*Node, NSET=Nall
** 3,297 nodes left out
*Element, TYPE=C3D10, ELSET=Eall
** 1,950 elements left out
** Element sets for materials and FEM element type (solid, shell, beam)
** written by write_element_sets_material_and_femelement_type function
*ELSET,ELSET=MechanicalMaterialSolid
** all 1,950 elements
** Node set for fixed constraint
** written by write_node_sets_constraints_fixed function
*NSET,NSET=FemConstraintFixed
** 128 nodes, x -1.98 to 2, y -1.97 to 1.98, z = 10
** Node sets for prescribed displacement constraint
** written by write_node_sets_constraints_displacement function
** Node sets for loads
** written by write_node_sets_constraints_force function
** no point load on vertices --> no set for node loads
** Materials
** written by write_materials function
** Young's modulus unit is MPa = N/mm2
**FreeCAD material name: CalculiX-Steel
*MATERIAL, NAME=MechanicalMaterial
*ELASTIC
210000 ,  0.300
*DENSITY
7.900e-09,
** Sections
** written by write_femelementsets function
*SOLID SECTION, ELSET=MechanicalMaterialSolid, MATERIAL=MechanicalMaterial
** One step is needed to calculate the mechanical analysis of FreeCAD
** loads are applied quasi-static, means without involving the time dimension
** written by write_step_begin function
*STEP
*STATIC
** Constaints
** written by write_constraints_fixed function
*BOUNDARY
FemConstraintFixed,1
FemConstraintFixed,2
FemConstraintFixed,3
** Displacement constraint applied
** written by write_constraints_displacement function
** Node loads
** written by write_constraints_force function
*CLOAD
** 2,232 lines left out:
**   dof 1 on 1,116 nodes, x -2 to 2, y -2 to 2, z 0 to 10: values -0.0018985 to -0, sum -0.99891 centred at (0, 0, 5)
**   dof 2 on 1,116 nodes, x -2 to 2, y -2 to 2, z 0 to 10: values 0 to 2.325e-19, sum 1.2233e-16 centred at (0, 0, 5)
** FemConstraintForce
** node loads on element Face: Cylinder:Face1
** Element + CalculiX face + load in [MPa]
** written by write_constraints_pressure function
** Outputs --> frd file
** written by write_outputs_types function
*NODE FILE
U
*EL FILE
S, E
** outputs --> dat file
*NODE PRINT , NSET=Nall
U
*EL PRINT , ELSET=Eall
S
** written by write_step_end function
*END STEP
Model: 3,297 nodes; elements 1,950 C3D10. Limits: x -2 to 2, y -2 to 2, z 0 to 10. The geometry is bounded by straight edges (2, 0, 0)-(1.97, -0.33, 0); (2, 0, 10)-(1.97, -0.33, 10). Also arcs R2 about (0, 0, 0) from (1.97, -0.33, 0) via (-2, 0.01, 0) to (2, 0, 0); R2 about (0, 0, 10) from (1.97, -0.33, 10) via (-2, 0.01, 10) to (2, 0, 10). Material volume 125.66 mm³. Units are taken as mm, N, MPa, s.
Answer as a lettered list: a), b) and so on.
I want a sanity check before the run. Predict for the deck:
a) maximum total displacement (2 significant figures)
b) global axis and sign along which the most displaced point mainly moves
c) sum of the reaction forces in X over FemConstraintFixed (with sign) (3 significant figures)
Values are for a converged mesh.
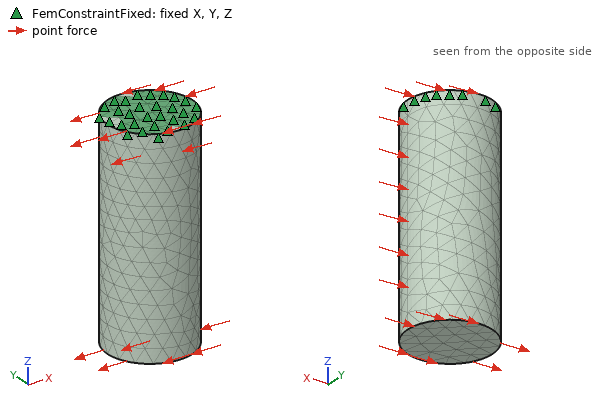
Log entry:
a) 5.4e-05 mm
b) -X
c) 0.999 N
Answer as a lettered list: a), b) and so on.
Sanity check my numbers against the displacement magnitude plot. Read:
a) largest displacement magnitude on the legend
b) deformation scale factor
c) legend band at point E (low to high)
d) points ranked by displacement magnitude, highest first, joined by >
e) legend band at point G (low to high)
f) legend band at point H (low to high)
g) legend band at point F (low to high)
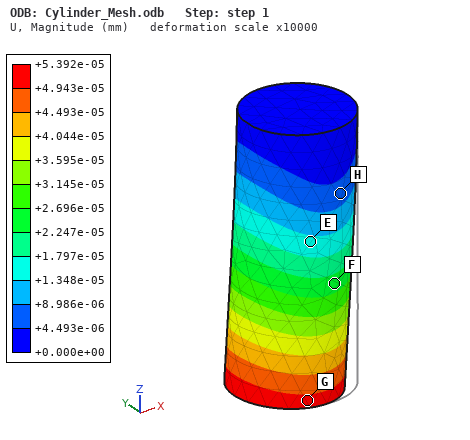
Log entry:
a) +5.392e-05 mm
b) 10000
c) +1.348e-05 to +1.797e-05 mm
d) G > F > E > H
e) +4.943e-05 to +5.392e-05 mm
f) +4.493e-06 to +8.986e-06 mm
g) +2.247e-05 to +2.696e-05 mm
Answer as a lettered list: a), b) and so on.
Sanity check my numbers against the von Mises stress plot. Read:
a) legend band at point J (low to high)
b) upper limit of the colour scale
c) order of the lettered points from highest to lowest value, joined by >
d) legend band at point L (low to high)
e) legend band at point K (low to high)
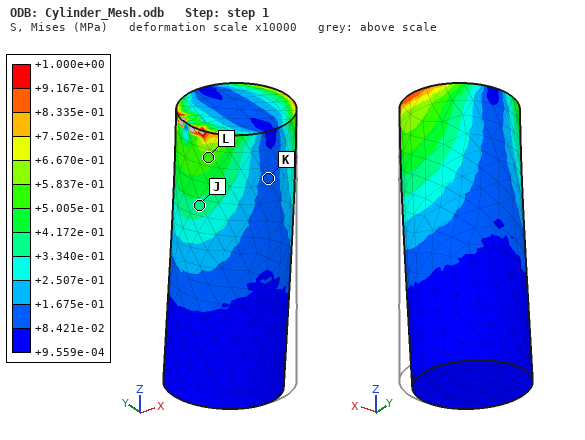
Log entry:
a) +3.340e-01 to +4.172e-01 MPa
b) +1.000e+00 MPa
c) L > J > K
d) +5.005e-01 to +5.837e-01 MPa
e) +8.421e-02 to +1.675e-01 MPa
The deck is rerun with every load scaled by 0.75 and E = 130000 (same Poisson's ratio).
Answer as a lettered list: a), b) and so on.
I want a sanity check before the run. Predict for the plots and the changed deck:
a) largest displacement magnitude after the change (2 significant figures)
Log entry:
a) 6.5e-05 mm
